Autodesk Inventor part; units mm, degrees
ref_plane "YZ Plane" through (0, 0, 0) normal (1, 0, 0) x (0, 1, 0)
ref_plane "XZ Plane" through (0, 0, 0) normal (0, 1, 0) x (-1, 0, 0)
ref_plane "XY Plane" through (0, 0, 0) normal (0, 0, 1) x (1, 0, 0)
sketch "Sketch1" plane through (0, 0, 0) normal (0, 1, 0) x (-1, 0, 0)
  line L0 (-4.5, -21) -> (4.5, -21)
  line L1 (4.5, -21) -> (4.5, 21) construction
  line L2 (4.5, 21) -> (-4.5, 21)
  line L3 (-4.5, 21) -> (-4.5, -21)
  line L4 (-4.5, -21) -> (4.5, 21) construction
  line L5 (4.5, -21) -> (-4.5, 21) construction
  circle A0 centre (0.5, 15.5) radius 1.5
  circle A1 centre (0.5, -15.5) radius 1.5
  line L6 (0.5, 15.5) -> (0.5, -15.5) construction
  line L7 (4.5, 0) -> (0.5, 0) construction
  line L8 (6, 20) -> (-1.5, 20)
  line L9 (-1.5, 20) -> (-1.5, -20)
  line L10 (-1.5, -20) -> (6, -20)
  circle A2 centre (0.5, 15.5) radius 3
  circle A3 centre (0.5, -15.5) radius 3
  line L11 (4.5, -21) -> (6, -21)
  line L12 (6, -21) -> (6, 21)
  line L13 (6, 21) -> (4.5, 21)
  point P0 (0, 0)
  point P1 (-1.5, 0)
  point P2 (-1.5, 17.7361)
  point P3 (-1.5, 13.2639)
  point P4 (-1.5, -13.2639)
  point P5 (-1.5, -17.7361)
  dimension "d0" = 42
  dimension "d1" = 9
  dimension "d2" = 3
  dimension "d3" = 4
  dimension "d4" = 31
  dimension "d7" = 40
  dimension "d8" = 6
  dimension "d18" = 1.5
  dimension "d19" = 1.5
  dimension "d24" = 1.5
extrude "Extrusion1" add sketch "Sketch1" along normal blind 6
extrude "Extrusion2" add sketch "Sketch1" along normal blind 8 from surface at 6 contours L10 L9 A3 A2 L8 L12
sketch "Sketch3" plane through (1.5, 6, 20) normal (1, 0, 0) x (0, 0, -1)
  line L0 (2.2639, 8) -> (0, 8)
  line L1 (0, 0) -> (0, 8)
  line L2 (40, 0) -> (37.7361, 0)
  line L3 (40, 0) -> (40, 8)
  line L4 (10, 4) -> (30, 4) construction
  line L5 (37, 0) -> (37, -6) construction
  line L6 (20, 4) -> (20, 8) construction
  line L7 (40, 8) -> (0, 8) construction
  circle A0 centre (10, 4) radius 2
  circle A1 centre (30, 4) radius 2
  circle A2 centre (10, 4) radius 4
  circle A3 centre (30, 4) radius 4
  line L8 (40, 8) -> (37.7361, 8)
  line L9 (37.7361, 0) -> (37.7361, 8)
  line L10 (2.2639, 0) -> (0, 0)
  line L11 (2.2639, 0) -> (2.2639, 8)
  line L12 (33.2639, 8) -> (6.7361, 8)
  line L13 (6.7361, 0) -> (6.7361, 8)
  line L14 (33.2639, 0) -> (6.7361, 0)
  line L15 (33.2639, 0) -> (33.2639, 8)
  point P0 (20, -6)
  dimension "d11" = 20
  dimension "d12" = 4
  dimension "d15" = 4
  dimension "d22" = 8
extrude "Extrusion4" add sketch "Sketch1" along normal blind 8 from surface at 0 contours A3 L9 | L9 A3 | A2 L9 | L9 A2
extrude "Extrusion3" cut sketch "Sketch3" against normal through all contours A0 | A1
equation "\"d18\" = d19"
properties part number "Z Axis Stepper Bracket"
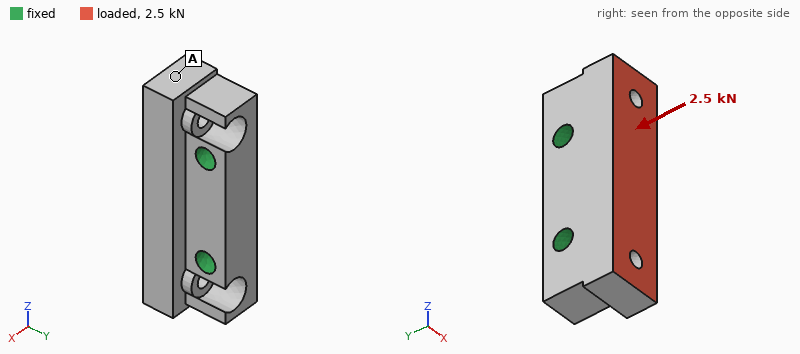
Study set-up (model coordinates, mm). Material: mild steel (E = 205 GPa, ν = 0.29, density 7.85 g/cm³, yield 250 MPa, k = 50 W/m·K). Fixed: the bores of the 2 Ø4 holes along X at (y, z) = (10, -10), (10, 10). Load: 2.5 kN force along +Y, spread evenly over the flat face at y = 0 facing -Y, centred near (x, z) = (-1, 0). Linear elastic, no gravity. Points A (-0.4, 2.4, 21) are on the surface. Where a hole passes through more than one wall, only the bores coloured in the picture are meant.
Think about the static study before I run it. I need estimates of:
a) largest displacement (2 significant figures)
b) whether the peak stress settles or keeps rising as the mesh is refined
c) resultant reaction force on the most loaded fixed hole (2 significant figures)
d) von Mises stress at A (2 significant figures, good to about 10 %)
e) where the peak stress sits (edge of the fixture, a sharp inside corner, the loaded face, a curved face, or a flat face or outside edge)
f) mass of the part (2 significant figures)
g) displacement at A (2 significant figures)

3.4 µm
keeps rising
1.3 kN
7.0 MPa
a sharp inside corner
35 g
2.4 µm
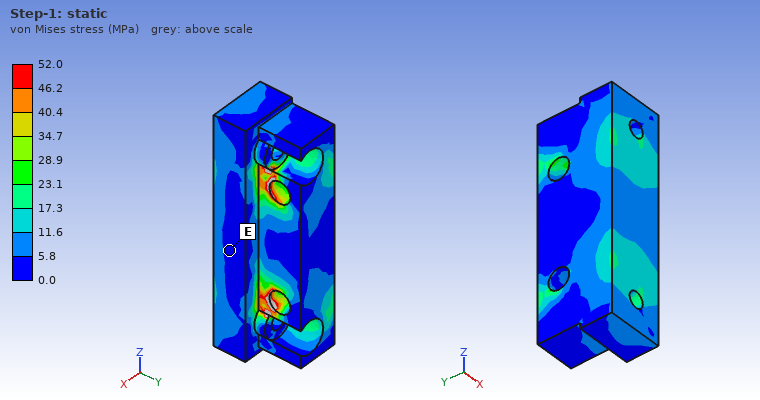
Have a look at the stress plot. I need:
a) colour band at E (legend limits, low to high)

0.0 to 5.8 MPa
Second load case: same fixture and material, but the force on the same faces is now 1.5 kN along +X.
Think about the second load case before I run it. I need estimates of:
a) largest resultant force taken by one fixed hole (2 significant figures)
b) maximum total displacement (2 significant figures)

750 N
5.4 µm
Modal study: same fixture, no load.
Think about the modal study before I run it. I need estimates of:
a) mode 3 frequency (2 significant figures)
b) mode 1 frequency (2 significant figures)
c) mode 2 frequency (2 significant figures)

33 kHz
27 kHz
27 kHz
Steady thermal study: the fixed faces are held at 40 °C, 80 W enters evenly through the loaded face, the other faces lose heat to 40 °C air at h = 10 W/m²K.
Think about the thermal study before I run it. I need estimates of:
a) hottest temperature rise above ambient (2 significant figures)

69 K
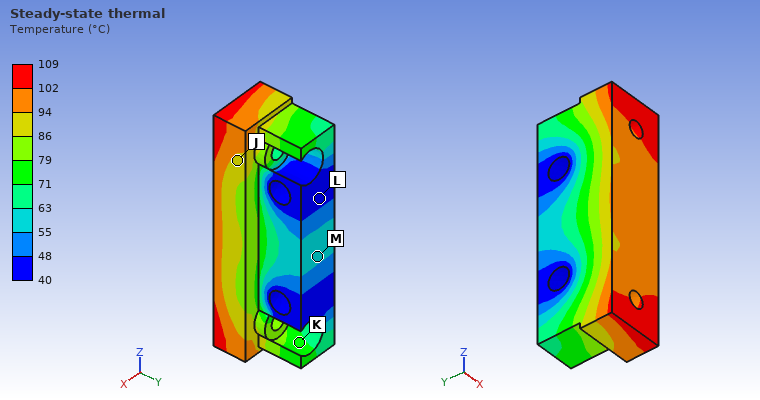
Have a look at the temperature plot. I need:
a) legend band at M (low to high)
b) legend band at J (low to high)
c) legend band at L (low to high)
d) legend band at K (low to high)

55 to 63 °C
86 to 94 °C
40 to 48 °C
71 to 79 °C
